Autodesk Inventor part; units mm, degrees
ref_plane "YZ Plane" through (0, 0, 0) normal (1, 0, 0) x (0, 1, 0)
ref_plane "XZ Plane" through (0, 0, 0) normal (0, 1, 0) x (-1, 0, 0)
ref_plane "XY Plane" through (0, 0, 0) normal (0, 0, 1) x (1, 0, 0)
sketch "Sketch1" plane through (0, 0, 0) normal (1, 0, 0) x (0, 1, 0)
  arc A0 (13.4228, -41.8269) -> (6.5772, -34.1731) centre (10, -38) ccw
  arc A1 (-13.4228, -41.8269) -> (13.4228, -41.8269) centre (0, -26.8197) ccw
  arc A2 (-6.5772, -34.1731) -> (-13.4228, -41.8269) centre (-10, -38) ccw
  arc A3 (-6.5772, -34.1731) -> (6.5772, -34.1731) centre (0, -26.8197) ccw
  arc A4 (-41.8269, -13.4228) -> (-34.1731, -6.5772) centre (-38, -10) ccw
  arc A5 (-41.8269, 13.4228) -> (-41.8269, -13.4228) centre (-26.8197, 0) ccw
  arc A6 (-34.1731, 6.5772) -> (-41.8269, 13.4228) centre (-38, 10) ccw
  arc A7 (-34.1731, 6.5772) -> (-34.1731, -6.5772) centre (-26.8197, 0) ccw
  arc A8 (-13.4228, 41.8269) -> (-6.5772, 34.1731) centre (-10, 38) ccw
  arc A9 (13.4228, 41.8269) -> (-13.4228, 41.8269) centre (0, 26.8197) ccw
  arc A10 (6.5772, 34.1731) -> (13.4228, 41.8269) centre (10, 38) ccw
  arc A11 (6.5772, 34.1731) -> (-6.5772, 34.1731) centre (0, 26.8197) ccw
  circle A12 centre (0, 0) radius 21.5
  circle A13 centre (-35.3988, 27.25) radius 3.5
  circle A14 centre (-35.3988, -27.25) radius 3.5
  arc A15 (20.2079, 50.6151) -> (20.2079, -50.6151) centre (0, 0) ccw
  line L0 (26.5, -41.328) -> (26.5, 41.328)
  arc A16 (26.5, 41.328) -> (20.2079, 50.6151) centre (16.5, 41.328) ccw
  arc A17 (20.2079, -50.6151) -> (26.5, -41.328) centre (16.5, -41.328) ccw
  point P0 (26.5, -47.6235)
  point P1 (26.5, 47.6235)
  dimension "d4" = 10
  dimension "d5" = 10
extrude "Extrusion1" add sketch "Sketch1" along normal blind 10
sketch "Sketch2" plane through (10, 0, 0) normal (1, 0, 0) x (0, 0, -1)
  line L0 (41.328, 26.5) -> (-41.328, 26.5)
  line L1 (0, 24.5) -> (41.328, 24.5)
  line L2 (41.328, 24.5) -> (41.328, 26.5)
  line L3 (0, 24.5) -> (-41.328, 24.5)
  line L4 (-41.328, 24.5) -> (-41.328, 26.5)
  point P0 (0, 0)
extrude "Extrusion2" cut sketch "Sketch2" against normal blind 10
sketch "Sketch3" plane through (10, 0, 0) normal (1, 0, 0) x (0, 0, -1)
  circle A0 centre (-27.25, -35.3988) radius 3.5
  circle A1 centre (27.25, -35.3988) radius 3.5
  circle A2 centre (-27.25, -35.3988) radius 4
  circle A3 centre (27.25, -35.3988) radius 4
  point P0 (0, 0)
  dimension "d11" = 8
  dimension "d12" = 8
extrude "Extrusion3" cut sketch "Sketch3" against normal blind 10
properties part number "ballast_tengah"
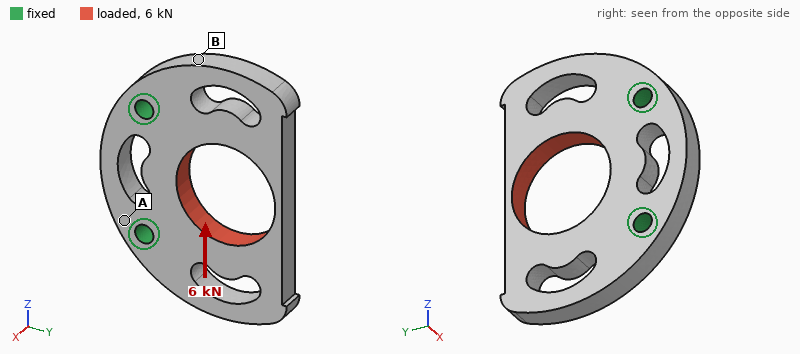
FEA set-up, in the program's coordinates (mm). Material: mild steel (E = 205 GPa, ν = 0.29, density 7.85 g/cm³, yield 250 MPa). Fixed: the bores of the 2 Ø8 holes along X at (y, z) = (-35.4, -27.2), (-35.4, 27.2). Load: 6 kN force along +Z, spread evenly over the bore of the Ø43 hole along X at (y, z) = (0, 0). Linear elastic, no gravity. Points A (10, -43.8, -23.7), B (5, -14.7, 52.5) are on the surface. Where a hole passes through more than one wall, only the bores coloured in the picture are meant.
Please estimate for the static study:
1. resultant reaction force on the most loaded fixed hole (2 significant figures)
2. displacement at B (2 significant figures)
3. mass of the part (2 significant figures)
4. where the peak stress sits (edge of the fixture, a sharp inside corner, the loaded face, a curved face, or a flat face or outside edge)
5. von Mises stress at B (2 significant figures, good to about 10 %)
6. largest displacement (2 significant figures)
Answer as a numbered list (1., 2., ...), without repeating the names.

1. 3.8 kN
2. 16 µm
3. 380 g
4. edge of the fixture
5. 28 MPa
6. 38 µm
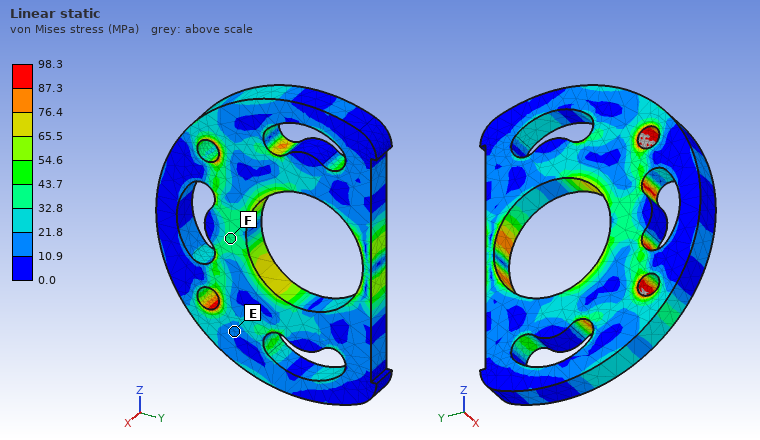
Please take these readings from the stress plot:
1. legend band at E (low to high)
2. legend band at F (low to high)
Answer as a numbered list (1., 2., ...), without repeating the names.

1. 10.9 to 21.8 MPa
2. 32.8 to 43.7 MPa
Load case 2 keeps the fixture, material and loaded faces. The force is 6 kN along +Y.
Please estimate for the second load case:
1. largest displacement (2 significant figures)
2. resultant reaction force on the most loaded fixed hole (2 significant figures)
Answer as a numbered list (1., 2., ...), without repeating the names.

1. 14 µm
2. 3.1 kN
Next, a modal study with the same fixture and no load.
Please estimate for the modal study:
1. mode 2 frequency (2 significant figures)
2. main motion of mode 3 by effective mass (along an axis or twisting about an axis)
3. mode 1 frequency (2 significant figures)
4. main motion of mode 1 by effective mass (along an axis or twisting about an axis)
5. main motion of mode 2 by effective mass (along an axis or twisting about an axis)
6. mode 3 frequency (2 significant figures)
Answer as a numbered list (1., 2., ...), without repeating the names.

1. 2800 Hz
2. along Z
3. 2000 Hz
4. along X
5. twisting about Y
6. 4400 Hz
